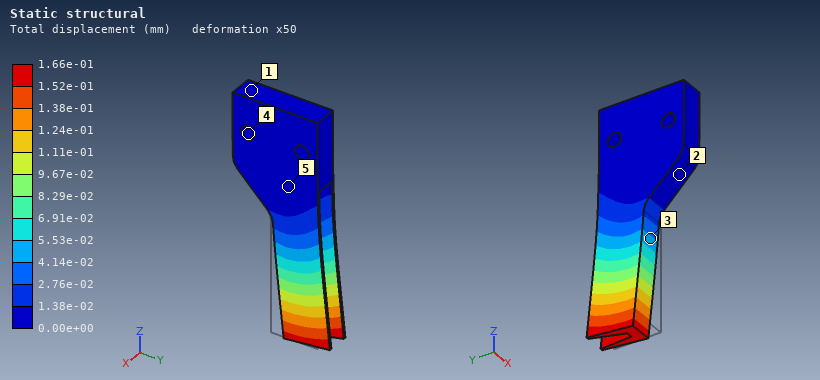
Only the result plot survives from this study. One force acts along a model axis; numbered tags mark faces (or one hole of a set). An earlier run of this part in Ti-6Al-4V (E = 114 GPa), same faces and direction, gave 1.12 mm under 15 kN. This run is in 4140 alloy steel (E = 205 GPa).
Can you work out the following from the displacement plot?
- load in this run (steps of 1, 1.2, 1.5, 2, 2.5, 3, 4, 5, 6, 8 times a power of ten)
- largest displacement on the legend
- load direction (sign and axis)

4 kN
1.66e-01 mm
+Y
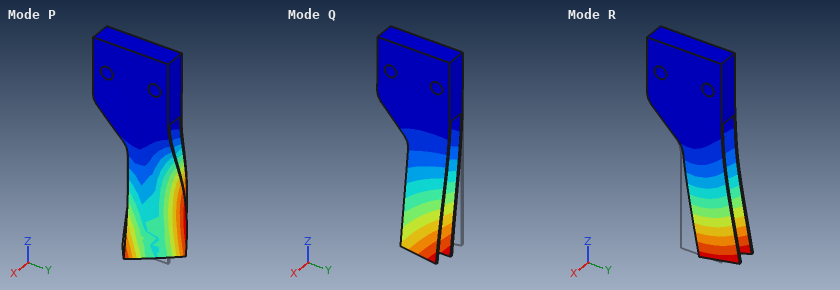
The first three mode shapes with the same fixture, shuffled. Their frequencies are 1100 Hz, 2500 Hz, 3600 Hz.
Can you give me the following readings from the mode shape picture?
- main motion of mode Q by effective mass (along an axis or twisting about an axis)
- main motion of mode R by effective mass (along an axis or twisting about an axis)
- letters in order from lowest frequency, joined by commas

along X
along Y
Q, R, P
